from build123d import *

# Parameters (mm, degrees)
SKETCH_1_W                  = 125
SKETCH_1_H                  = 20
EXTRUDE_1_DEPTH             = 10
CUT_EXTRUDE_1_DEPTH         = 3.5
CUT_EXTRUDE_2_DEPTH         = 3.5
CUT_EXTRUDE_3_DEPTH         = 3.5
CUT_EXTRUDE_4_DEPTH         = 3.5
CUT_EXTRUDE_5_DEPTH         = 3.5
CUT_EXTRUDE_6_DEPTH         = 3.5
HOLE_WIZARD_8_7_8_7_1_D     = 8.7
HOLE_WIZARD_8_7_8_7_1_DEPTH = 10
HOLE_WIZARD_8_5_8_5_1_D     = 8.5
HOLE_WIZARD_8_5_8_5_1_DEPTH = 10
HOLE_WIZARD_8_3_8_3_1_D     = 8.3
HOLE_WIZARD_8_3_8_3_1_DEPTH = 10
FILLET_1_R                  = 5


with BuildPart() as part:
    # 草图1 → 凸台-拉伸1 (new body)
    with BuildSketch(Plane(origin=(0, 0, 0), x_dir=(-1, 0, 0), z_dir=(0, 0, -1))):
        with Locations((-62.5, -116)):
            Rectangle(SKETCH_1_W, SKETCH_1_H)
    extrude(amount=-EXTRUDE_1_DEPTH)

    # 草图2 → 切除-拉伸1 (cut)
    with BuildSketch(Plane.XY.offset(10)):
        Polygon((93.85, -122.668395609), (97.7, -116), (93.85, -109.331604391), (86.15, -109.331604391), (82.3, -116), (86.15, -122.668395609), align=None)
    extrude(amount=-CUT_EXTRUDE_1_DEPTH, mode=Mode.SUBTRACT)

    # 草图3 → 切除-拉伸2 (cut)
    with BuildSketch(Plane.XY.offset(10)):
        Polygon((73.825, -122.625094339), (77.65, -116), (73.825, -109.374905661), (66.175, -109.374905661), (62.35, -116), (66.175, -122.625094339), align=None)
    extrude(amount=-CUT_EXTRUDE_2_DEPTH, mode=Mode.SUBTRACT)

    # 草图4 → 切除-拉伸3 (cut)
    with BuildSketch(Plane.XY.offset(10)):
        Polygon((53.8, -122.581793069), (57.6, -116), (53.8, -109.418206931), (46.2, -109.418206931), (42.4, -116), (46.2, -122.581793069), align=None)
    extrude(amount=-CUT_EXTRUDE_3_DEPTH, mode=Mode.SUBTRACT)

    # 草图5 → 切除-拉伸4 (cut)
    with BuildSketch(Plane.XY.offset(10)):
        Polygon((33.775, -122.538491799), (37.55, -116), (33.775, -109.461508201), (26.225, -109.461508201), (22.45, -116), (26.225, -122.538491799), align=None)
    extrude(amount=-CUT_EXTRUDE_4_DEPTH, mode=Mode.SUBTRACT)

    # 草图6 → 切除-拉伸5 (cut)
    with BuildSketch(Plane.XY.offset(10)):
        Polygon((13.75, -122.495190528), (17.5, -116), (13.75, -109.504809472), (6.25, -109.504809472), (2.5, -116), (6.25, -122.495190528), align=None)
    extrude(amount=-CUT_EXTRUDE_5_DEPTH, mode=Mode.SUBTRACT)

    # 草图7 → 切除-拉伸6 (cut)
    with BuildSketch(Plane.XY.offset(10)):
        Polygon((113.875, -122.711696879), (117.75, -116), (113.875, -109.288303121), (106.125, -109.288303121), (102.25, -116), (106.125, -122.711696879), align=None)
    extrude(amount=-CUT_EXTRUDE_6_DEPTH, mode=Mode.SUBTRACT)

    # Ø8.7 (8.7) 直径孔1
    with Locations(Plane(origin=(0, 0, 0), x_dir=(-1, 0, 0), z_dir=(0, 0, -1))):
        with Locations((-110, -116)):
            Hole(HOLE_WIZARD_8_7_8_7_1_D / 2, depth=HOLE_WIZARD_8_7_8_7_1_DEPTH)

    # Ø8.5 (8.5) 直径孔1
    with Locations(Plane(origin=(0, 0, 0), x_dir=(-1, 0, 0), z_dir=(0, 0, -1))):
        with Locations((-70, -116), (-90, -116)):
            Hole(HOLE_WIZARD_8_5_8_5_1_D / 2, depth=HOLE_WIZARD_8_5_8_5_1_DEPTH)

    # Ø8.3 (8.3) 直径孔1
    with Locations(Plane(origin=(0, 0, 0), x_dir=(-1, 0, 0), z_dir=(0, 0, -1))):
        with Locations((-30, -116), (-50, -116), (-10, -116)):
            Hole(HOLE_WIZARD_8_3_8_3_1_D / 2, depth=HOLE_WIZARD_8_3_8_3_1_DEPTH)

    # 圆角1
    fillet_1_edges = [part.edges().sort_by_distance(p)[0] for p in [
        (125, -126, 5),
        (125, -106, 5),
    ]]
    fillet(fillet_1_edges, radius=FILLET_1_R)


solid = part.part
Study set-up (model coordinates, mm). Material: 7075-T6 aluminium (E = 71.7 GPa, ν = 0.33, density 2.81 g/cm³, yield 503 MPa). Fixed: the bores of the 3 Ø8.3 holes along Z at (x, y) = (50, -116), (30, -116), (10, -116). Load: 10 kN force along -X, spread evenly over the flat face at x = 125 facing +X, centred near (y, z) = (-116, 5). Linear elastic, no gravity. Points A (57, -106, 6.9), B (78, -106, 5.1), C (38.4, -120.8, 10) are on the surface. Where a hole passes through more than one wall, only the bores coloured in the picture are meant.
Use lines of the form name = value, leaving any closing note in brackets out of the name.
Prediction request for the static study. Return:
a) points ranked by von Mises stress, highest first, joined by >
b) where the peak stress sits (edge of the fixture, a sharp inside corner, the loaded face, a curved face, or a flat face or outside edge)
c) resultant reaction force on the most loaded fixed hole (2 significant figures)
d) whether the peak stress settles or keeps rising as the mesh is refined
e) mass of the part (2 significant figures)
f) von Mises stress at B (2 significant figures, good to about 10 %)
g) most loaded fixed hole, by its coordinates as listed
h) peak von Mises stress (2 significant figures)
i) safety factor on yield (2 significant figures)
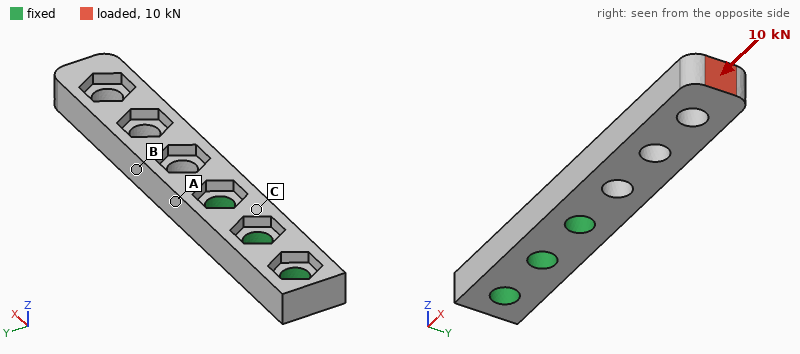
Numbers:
points ranked by von Mises stress, highest first, joined by > = B > A > C
where the peak stress sits = a curved face
resultant reaction force on the most loaded fixed hole = 8.6 kN
whether the peak stress settles or keeps rising as the mesh is refined = settles
mass of the part = 55 g
von Mises stress at B = 110 MPa
most loaded fixed hole, by its coordinates as listed = (50, -116)
peak von Mises stress = 290 MPa
safety factor on yield = 1.8
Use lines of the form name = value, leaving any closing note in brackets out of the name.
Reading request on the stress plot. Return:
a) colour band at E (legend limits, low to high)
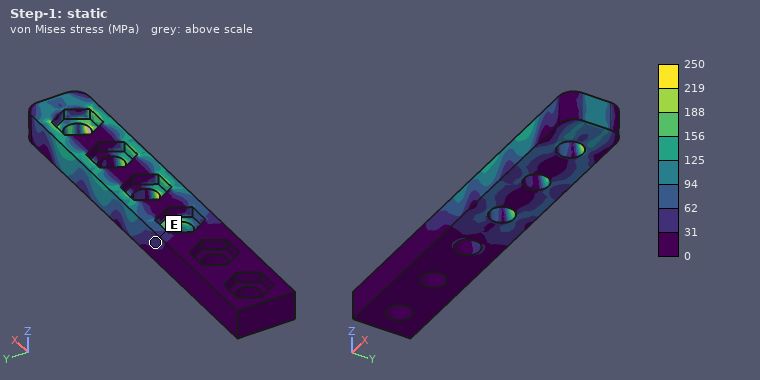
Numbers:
colour band at E = 31 to 62 MPa
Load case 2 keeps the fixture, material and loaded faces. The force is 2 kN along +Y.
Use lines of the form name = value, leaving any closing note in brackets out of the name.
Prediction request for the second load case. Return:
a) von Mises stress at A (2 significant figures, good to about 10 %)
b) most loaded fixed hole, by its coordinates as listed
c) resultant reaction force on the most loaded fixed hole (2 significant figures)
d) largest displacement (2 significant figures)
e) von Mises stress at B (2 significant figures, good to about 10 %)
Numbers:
von Mises stress at A = 210 MPa
most loaded fixed hole, by its coordinates as listed = (50, -116)
resultant reaction force on the most loaded fixed hole = 4.7 kN
largest displacement = 0.87 mm
von Mises stress at B = 150 MPa
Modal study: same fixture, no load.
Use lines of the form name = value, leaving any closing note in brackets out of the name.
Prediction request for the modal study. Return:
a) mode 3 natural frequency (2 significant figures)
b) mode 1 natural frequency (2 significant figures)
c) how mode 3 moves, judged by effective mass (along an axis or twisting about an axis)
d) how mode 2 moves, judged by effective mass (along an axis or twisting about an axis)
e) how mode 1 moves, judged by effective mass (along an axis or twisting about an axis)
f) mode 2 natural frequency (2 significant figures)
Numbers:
mode 3 natural frequency = 5900 Hz
mode 1 natural frequency = 1200 Hz
how mode 3 moves, judged by effective mass = twisting about X
how mode 2 moves, judged by effective mass = along Y
how mode 1 moves, judged by effective mass = along Z
mode 2 natural frequency = 2600 Hz
